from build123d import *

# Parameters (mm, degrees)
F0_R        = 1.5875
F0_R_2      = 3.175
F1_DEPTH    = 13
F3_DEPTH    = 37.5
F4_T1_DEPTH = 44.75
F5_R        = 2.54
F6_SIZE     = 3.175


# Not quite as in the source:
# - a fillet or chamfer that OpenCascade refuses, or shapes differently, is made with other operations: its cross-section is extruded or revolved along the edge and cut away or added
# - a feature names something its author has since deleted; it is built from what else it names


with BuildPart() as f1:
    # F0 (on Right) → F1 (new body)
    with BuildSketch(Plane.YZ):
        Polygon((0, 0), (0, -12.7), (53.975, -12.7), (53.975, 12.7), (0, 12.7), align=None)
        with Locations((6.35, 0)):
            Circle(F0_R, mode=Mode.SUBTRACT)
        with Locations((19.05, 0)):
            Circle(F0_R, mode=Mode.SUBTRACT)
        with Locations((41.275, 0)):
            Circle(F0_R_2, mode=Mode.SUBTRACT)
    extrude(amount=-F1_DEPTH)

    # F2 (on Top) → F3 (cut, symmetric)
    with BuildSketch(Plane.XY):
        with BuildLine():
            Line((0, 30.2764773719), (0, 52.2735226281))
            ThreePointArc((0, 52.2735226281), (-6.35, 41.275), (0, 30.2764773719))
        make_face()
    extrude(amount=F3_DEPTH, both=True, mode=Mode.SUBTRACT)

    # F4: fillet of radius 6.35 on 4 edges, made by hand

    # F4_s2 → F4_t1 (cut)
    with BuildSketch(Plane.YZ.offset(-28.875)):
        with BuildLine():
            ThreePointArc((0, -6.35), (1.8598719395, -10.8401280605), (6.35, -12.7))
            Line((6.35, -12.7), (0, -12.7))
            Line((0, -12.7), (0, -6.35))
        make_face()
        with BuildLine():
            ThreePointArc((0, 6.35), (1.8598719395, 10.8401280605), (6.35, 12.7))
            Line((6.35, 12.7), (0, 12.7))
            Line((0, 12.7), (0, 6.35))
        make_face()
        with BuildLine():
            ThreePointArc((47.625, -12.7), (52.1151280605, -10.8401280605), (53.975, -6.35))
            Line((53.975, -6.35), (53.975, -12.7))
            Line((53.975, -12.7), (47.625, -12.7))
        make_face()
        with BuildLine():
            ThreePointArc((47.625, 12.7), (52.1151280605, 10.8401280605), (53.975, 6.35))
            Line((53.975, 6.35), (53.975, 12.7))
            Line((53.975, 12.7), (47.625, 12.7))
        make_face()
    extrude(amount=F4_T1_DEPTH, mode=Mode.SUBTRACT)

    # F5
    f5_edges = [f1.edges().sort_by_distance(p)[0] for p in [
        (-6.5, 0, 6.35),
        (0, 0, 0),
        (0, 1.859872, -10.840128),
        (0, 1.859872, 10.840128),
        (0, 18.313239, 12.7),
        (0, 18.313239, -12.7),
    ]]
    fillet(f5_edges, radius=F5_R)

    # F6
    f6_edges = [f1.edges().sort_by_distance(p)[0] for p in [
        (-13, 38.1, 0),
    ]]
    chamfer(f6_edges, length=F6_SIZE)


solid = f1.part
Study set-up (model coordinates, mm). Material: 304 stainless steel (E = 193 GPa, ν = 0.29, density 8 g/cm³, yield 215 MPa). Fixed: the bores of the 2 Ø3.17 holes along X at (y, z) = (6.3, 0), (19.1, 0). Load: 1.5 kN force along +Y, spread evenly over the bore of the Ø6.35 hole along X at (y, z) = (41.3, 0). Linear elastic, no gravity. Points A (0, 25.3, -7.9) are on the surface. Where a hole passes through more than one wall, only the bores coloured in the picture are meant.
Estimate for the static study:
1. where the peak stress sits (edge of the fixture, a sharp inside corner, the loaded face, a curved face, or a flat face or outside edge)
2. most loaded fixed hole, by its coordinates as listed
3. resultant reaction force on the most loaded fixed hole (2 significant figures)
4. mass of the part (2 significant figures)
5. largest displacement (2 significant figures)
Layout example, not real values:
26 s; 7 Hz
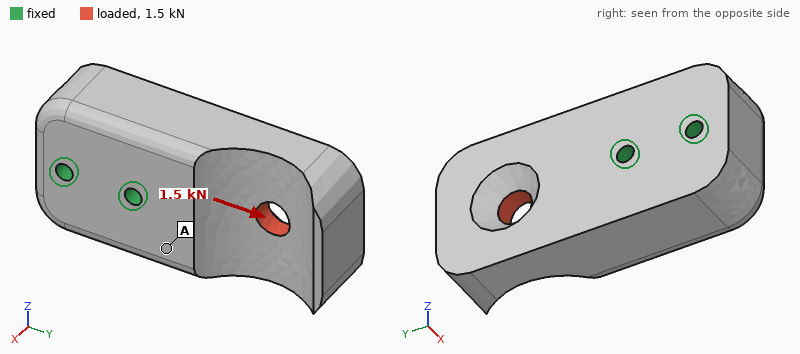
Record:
the loaded face; (19.1, 0); 1.1 kN; 110 g; 2.5 µm
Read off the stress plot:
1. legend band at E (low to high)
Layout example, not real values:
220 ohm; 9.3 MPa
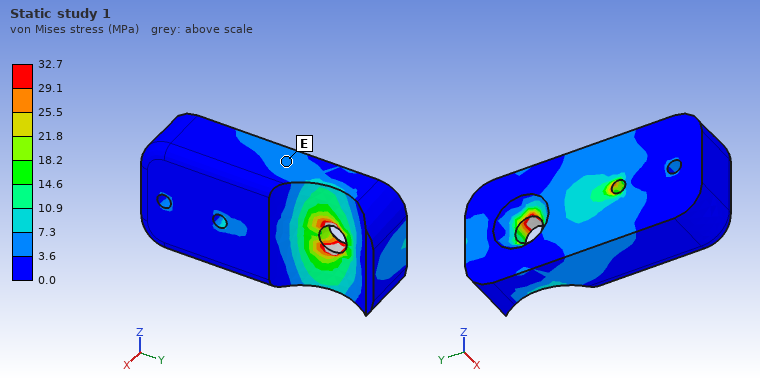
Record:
3.6 to 7.3 MPa
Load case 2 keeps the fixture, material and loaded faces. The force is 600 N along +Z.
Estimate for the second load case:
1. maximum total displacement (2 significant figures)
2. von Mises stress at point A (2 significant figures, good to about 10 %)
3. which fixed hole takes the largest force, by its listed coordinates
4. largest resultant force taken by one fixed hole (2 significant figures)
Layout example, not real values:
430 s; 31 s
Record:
5.2 µm; 3.7 MPa; (19.1, 0); 1.4 kN
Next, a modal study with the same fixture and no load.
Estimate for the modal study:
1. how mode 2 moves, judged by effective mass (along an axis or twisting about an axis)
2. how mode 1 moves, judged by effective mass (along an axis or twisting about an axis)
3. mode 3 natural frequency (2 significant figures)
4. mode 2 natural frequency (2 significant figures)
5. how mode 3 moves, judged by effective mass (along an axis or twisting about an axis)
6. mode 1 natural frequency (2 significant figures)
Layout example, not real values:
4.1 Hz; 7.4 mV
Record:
along Z; along X; 14 kHz; 9400 Hz; twisting about Y; 6500 Hz
